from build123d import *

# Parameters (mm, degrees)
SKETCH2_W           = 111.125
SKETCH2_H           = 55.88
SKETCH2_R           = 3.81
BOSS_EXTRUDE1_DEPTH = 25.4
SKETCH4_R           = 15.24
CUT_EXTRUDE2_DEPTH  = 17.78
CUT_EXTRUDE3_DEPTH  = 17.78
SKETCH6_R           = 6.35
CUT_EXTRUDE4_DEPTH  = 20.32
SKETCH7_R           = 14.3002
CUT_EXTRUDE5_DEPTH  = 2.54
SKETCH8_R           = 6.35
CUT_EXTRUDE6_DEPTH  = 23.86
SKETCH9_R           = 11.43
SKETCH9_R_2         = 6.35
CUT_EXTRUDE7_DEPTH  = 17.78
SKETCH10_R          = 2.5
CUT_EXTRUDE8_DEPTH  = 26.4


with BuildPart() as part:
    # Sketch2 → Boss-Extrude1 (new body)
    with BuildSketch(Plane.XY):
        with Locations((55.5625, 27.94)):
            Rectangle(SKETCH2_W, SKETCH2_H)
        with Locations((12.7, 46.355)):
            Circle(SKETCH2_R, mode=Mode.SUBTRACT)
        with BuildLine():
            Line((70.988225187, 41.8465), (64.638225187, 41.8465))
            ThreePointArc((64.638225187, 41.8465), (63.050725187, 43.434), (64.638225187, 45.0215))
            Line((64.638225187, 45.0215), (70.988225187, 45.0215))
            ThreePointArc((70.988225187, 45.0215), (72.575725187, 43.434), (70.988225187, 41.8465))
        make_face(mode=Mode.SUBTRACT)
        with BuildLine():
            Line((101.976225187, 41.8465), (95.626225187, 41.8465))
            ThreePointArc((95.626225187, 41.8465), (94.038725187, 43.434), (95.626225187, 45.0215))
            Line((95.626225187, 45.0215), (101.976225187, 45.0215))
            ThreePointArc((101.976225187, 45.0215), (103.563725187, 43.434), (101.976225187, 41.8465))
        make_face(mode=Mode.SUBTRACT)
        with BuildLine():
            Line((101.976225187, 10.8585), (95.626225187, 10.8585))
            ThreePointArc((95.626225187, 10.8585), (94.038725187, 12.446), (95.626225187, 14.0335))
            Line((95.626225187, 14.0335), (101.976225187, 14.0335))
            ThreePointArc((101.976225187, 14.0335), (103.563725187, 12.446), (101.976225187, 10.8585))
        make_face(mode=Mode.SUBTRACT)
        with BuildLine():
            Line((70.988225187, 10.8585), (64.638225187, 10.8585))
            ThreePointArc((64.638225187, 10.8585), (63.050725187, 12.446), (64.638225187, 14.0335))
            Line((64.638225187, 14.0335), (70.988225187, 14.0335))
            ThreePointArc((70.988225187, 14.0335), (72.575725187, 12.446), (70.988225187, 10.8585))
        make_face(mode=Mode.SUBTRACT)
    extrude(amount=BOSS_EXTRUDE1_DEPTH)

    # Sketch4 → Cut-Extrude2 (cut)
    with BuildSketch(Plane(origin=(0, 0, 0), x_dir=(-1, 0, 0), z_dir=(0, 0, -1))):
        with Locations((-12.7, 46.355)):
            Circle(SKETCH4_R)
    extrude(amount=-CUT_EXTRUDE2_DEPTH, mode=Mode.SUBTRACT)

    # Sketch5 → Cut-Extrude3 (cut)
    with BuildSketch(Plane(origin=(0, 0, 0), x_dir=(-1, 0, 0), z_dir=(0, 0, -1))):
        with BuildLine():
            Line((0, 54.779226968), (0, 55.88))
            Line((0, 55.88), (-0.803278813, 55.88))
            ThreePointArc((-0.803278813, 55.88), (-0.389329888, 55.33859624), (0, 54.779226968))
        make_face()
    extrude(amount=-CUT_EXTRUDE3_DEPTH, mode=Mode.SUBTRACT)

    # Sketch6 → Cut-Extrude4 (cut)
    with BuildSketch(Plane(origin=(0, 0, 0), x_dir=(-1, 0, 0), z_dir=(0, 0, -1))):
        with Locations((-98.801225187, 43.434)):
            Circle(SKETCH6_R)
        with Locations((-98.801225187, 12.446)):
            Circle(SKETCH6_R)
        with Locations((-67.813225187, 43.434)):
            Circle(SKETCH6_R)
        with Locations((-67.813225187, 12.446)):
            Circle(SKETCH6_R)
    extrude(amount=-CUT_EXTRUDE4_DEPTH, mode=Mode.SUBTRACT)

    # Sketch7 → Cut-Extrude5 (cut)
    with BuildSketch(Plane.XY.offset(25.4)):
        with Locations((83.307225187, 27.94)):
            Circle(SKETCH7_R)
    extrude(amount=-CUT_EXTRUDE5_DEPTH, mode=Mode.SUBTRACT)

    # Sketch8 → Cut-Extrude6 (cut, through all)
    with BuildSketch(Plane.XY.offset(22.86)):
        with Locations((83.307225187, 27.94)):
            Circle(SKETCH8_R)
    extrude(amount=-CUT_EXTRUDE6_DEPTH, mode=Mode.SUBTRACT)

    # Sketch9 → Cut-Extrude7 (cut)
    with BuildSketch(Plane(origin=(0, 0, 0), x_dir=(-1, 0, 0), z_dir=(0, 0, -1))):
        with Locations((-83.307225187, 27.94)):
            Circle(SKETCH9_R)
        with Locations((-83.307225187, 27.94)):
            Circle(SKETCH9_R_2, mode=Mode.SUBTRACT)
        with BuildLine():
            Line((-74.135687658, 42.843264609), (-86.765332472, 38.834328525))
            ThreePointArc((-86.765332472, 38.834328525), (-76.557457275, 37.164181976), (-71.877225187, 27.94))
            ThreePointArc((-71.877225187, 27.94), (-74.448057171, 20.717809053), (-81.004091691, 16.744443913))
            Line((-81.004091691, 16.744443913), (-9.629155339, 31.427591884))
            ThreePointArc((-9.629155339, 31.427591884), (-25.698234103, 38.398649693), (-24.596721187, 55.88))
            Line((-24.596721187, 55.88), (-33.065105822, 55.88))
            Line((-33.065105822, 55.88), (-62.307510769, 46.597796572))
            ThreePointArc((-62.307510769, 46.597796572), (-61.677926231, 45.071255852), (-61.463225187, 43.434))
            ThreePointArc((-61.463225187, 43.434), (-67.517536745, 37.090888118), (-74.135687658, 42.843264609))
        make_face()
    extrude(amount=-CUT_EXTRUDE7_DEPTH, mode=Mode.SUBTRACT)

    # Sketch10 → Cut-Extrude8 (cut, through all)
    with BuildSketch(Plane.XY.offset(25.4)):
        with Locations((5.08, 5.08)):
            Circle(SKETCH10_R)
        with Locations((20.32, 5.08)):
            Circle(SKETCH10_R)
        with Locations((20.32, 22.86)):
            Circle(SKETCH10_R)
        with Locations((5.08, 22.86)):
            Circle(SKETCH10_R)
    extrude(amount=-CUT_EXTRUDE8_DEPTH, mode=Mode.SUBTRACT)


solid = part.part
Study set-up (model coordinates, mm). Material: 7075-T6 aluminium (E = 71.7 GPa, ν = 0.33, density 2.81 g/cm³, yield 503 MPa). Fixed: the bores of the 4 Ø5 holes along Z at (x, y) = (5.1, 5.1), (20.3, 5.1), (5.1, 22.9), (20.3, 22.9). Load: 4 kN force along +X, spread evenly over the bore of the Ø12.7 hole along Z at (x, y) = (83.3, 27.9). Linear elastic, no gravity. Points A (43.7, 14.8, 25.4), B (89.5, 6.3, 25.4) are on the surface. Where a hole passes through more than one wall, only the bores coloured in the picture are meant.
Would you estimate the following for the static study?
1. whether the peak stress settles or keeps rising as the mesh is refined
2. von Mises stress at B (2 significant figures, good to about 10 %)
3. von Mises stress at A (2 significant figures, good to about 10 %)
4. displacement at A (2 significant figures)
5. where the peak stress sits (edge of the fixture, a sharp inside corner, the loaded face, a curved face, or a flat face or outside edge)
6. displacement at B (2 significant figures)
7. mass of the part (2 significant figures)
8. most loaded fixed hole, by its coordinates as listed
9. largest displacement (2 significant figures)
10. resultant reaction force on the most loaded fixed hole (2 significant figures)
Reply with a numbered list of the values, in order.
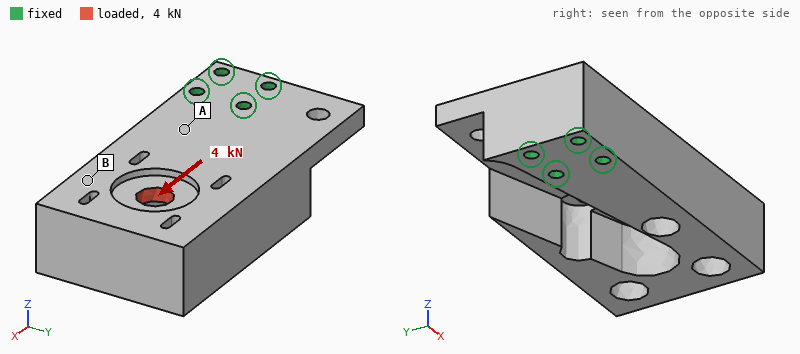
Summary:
1. keeps rising
2. 3.7 MPa
3. 9.0 MPa
4. 4.6 µm
5. edge of the fixture
6. 19 µm
7. 280 g
8. (20.3, 22.9)
9. 29 µm
10. 3.2 kN
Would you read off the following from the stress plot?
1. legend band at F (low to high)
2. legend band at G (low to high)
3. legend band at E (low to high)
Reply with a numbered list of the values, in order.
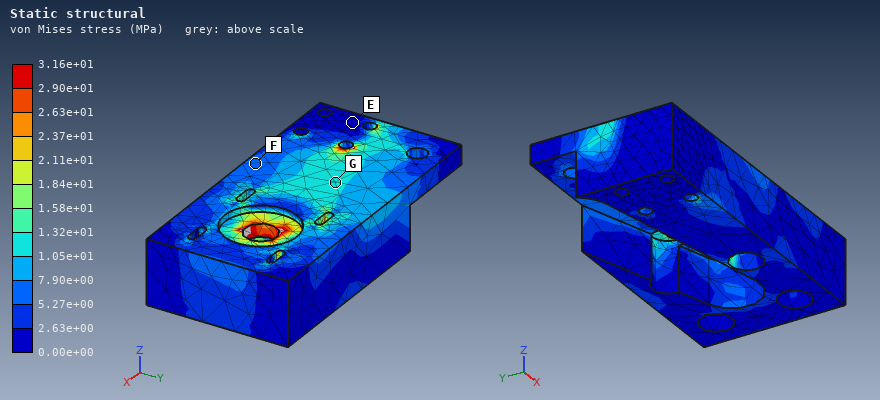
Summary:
1. 5.27e+00 to 7.90e+00 MPa
2. 1.05e+01 to 1.32e+01 MPa
3. 0.00e+00 to 2.63e+00 MPa
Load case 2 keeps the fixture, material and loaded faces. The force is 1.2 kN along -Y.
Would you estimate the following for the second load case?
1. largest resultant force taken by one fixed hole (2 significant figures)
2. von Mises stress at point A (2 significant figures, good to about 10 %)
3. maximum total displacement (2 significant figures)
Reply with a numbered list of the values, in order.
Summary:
1. 2.9 kN
2. 8.9 MPa
3. 43 µm
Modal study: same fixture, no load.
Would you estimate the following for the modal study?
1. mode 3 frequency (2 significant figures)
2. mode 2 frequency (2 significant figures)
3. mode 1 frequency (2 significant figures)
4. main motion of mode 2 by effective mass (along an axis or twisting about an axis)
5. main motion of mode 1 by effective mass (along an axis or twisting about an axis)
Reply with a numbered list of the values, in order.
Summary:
1. 3600 Hz
2. 2600 Hz
3. 1500 Hz
4. along Y
5. along Z
